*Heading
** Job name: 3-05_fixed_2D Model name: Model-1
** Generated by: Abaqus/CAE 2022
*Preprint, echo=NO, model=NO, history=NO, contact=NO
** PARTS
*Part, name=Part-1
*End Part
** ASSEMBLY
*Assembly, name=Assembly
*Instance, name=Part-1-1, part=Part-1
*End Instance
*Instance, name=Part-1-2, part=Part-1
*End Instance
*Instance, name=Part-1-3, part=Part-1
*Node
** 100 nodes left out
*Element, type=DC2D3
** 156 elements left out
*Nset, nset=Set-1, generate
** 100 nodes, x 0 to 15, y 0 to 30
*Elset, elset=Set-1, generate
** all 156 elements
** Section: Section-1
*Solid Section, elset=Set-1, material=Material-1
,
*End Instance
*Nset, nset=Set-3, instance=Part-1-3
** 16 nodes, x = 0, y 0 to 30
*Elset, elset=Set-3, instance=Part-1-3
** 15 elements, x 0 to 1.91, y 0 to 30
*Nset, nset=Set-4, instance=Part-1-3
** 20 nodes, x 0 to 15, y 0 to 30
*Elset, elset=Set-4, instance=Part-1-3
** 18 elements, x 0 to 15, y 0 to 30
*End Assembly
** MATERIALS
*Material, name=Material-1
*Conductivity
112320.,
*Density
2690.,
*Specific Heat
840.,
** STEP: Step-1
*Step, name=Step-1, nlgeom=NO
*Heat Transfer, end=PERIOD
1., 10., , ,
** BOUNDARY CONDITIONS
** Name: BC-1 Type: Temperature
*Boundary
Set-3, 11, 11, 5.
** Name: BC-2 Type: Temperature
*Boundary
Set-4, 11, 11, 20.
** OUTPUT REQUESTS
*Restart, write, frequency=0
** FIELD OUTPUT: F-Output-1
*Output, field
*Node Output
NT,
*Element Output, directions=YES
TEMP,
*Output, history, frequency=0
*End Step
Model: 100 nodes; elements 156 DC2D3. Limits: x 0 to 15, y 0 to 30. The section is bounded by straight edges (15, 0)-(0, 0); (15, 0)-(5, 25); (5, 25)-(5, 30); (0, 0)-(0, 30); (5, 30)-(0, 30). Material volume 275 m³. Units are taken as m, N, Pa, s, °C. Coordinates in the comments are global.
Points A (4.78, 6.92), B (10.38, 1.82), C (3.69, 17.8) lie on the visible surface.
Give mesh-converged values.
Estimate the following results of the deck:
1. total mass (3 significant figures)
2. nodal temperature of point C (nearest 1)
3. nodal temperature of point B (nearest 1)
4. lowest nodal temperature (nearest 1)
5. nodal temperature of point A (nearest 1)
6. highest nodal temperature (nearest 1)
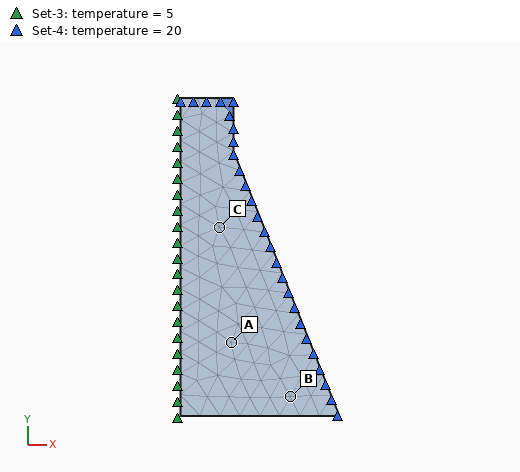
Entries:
7.40e+05 kg
0 °C
0 °C
0 °C
0 °C
20 °C
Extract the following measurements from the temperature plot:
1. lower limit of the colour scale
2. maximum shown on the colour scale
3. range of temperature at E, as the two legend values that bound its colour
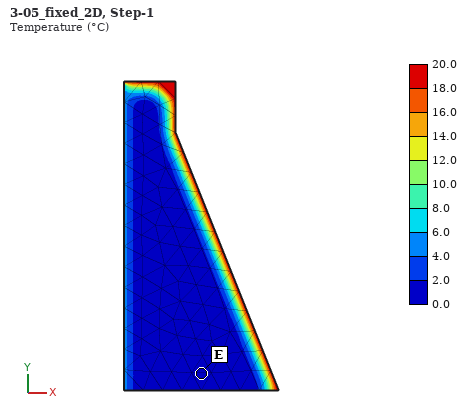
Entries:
0.0 °C
20.0 °C
0.0 to 2.0 °C
